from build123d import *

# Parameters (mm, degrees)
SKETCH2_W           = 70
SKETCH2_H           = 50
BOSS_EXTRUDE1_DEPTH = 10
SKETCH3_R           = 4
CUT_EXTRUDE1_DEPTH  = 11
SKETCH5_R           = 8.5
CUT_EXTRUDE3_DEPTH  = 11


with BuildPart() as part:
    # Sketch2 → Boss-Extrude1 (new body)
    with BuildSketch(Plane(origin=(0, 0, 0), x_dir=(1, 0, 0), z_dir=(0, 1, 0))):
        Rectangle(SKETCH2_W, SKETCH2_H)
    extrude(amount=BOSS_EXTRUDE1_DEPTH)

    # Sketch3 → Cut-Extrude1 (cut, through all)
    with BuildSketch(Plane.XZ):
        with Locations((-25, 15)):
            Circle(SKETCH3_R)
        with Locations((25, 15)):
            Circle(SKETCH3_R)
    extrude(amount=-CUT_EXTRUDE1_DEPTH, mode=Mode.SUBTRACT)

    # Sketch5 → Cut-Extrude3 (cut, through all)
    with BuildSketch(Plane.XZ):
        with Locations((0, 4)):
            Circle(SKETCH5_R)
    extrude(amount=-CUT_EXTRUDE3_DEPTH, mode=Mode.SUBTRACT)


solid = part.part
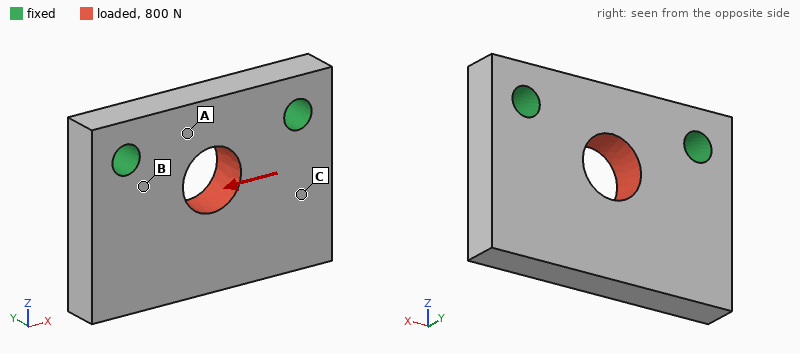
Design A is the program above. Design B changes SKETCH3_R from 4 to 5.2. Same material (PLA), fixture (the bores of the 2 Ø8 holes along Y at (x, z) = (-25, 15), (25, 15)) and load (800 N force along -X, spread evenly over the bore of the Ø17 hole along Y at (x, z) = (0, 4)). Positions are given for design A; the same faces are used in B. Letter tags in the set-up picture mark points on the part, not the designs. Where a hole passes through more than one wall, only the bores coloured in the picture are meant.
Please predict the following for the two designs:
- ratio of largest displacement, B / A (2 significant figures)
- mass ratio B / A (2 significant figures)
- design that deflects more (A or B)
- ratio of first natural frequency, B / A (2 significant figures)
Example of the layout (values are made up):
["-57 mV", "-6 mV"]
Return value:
["0.90", "0.98", "A", "1.1"]
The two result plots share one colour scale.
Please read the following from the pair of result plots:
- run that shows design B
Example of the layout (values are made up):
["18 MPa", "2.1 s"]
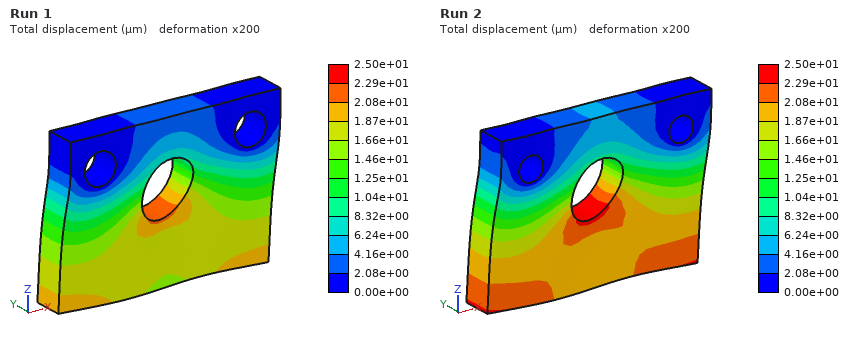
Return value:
["Run 1"]
